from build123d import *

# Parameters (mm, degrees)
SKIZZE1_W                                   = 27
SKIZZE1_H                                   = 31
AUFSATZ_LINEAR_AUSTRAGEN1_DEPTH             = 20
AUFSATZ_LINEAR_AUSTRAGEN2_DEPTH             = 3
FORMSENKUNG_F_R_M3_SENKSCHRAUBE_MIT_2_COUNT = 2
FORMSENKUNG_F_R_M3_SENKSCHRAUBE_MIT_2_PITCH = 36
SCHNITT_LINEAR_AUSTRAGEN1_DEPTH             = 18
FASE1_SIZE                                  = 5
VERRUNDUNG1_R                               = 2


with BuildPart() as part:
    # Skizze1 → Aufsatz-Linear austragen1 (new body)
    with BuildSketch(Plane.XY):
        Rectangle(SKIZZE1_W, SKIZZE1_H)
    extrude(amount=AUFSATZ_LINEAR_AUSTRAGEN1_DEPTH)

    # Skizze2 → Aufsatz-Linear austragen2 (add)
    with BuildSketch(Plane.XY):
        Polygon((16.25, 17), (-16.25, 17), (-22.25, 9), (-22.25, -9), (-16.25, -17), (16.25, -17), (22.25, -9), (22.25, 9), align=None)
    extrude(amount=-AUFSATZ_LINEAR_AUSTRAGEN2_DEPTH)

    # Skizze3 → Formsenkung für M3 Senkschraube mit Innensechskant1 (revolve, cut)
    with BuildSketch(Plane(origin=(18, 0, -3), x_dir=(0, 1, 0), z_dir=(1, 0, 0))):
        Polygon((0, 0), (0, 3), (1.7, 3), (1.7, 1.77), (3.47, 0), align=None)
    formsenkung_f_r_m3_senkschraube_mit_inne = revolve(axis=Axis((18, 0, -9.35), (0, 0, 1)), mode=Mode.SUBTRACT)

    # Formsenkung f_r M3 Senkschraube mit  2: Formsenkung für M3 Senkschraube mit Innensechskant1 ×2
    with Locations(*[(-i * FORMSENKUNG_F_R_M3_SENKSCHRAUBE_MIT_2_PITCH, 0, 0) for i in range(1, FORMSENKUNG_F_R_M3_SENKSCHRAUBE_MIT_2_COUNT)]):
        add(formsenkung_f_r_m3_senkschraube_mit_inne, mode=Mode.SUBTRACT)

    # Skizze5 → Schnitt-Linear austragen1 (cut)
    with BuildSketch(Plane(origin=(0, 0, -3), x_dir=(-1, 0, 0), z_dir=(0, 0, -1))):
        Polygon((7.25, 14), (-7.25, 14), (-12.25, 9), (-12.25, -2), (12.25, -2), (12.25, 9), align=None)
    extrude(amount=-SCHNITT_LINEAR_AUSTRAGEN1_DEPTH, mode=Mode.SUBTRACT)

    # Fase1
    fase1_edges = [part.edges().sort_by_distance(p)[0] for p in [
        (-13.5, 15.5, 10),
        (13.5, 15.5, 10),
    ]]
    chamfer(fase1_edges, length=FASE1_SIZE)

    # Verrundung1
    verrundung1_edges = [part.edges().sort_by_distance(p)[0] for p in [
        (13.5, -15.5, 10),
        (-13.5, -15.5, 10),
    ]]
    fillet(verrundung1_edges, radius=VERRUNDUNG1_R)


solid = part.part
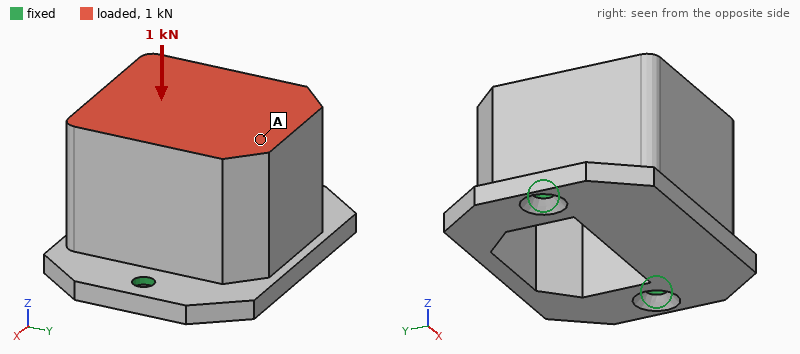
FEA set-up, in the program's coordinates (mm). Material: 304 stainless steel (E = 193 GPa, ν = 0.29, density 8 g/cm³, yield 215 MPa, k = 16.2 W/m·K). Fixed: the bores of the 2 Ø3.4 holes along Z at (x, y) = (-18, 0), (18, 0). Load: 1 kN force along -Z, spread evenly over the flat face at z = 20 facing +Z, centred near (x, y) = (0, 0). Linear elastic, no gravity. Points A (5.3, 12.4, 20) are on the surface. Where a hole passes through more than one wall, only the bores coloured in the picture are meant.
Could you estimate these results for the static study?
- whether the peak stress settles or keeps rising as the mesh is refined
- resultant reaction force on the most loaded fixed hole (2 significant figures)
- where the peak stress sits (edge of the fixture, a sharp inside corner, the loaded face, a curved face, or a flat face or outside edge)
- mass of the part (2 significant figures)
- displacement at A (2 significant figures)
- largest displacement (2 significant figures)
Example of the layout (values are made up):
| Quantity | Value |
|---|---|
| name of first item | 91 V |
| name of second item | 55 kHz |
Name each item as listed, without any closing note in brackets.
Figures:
| Quantity | Value |
|---|---|
| whether the peak stress settles or keeps rising as the mesh is refined | keeps rising |
| resultant reaction force on the most loaded fixed hole | 500 N |
| where the peak stress sits | edge of the fixture |
| mass of the part | 110 g |
| displacement at A | 6.2 µm |
| largest displacement | 6.4 µm |
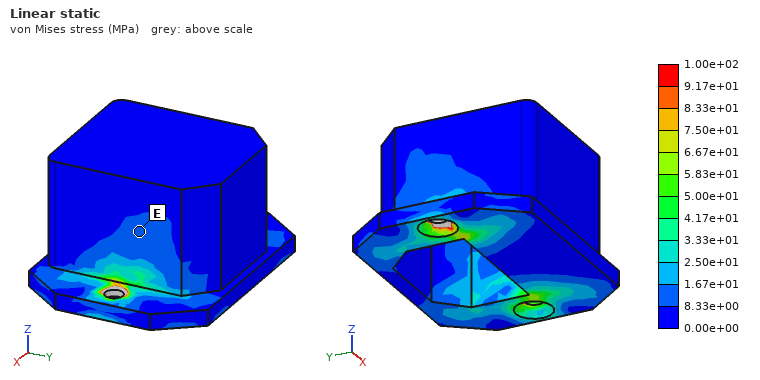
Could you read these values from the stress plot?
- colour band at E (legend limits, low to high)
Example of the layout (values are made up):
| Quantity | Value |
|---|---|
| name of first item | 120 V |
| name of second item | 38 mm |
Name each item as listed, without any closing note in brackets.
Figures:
| Quantity | Value |
|---|---|
| colour band at E | 8.33e+00 to 1.67e+01 MPa |
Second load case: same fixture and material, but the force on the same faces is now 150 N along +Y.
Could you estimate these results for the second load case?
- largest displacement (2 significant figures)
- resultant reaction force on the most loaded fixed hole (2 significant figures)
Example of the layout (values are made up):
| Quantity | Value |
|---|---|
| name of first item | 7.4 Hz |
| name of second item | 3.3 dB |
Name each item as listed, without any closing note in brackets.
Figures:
| Quantity | Value |
|---|---|
| largest displacement | 37 µm |
| resultant reaction force on the most loaded fixed hole | 76 N |
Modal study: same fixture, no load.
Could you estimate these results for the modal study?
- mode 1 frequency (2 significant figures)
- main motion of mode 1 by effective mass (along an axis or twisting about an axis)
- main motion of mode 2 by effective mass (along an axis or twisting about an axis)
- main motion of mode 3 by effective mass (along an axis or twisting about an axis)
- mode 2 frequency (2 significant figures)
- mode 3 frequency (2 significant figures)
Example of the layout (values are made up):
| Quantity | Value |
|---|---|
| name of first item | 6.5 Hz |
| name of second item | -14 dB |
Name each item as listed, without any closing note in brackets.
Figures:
| Quantity | Value |
|---|---|
| mode 1 frequency | 1500 Hz |
| main motion of mode 1 by effective mass | along Y |
| main motion of mode 2 by effective mass | along X |
| main motion of mode 3 by effective mass | along Z |
| mode 2 frequency | 6300 Hz |
| mode 3 frequency | 6600 Hz |
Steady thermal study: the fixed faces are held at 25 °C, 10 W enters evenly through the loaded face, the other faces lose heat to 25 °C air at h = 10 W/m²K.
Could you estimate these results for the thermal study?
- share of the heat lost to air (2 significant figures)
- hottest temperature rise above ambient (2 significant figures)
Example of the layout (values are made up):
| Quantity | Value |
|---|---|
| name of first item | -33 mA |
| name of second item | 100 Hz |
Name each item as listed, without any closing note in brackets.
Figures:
| Quantity | Value |
|---|---|
| share of the heat lost to air | 29 % |
| hottest temperature rise above ambient | 76 K |
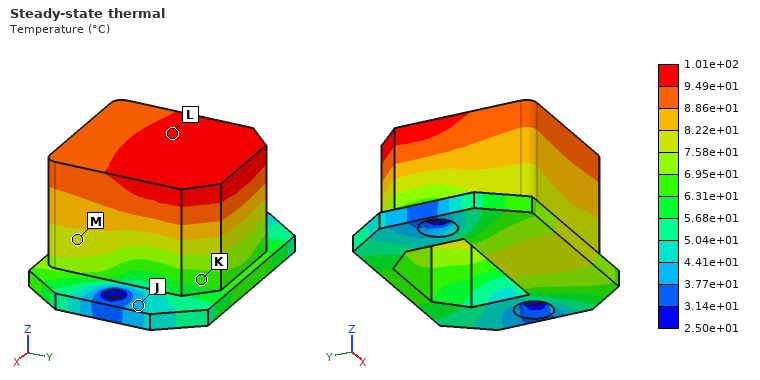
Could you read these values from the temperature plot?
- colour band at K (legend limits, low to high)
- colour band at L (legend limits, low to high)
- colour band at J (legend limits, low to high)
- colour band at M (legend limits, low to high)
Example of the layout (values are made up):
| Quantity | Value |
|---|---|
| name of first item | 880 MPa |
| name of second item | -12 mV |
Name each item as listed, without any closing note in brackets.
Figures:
| Quantity | Value |
|---|---|
| colour band at K | 6.31e+01 to 6.95e+01 °C |
| colour band at L | 9.49e+01 to 1.01e+02 °C |
| colour band at J | 3.77e+01 to 4.41e+01 °C |
| colour band at M | 7.58e+01 to 8.22e+01 °C |
